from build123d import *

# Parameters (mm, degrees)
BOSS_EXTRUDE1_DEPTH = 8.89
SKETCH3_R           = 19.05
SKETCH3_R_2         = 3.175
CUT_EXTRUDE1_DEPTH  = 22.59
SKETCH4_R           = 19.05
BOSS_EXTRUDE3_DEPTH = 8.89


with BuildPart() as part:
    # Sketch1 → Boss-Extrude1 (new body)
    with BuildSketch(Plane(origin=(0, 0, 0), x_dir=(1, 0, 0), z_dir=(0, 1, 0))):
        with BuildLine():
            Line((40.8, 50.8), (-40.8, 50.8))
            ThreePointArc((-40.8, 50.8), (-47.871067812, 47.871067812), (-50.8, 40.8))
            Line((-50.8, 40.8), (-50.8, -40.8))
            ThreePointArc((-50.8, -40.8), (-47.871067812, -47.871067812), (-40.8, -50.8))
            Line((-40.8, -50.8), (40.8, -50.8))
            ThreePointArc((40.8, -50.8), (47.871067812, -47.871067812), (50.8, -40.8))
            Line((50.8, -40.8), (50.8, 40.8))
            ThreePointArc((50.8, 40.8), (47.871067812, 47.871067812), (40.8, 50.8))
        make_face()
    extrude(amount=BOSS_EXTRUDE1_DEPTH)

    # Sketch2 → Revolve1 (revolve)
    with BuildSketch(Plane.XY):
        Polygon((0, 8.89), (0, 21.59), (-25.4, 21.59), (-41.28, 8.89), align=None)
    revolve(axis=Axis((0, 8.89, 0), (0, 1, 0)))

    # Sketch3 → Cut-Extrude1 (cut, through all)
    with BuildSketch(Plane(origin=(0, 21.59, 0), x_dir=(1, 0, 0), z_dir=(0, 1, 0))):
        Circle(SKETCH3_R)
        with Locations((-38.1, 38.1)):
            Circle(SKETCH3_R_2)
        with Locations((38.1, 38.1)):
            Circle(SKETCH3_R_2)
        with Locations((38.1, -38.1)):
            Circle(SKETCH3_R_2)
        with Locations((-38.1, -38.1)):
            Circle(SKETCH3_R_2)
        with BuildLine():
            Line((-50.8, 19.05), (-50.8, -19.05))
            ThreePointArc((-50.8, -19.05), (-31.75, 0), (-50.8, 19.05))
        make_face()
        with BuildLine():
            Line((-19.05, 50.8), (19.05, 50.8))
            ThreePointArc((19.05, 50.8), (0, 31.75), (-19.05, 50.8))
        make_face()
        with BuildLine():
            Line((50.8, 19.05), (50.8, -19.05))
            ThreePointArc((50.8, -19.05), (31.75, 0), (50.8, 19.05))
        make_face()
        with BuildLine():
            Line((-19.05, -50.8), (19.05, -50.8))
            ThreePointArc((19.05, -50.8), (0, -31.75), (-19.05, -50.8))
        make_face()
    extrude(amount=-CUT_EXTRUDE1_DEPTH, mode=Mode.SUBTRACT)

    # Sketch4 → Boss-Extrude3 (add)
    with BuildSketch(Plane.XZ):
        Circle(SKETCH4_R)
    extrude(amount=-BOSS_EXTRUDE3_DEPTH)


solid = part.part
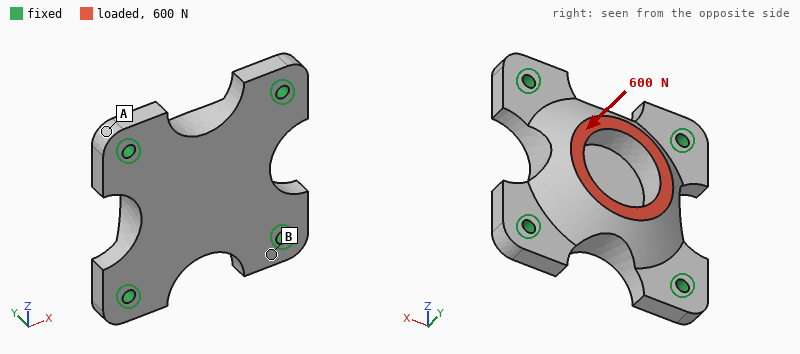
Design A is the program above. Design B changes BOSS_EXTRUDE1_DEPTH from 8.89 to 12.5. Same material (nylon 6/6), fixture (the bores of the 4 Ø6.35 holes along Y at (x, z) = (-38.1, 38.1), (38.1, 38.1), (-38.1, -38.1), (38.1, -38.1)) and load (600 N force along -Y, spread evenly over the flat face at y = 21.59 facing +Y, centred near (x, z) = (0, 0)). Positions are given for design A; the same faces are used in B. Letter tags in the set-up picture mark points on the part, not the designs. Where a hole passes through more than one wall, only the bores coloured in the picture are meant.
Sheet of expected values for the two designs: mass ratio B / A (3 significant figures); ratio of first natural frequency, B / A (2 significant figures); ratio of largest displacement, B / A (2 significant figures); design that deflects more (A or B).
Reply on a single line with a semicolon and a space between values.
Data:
1.13; 1.2; 0.78; A
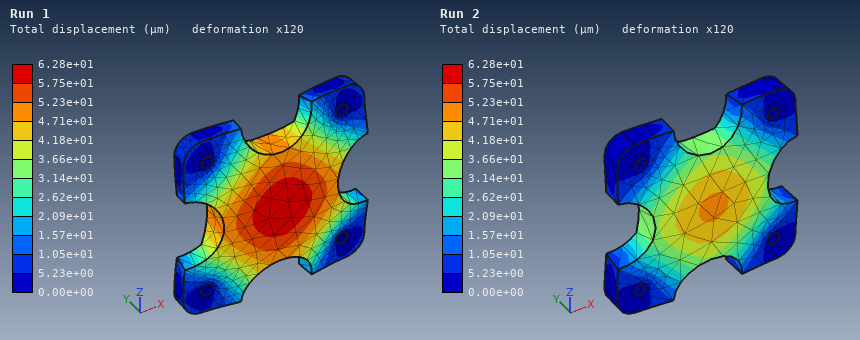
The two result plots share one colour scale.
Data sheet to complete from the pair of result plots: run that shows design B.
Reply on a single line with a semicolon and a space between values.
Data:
Run 2
